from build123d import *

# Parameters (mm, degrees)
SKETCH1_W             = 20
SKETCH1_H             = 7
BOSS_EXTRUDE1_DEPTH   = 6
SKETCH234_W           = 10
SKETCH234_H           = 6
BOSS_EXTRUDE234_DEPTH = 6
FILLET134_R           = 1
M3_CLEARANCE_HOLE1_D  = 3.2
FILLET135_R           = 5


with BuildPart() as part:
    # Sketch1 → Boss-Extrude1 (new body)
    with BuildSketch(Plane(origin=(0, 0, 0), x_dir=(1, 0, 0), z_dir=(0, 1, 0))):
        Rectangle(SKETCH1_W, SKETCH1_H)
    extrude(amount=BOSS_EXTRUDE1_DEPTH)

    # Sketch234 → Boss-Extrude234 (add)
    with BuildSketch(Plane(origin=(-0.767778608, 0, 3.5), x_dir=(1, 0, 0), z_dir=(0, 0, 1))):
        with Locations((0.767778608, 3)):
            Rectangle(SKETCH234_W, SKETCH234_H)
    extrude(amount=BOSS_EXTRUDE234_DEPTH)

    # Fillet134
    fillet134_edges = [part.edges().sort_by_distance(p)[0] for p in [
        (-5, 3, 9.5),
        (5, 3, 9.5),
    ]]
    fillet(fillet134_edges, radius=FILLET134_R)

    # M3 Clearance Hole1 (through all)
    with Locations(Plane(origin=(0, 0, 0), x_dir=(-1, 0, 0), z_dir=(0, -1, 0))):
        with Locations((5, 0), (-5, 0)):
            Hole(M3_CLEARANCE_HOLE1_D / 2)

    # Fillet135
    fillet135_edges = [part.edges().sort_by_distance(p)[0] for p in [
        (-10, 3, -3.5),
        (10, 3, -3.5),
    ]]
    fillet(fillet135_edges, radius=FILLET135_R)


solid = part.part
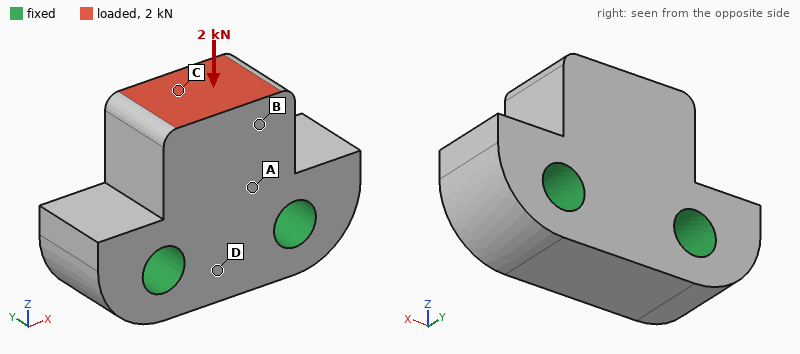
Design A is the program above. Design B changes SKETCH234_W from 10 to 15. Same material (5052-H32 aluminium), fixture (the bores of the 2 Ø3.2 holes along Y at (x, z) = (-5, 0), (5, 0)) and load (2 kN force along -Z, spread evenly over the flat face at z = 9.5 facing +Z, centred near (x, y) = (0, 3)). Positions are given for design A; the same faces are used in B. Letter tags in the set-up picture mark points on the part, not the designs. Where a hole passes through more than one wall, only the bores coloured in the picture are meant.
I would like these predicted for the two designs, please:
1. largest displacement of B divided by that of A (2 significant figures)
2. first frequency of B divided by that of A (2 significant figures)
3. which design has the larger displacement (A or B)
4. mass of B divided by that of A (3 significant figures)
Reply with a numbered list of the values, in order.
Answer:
1. 0.66
2. 1.0
3. A
4. 1.17
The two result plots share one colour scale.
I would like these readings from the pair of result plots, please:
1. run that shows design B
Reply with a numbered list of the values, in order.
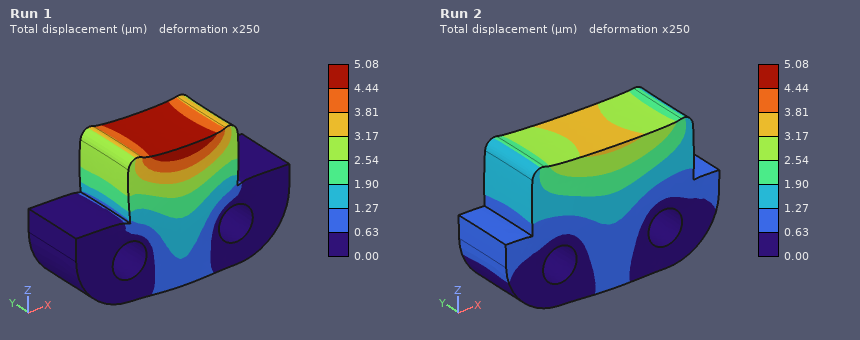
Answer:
1. Run 2
